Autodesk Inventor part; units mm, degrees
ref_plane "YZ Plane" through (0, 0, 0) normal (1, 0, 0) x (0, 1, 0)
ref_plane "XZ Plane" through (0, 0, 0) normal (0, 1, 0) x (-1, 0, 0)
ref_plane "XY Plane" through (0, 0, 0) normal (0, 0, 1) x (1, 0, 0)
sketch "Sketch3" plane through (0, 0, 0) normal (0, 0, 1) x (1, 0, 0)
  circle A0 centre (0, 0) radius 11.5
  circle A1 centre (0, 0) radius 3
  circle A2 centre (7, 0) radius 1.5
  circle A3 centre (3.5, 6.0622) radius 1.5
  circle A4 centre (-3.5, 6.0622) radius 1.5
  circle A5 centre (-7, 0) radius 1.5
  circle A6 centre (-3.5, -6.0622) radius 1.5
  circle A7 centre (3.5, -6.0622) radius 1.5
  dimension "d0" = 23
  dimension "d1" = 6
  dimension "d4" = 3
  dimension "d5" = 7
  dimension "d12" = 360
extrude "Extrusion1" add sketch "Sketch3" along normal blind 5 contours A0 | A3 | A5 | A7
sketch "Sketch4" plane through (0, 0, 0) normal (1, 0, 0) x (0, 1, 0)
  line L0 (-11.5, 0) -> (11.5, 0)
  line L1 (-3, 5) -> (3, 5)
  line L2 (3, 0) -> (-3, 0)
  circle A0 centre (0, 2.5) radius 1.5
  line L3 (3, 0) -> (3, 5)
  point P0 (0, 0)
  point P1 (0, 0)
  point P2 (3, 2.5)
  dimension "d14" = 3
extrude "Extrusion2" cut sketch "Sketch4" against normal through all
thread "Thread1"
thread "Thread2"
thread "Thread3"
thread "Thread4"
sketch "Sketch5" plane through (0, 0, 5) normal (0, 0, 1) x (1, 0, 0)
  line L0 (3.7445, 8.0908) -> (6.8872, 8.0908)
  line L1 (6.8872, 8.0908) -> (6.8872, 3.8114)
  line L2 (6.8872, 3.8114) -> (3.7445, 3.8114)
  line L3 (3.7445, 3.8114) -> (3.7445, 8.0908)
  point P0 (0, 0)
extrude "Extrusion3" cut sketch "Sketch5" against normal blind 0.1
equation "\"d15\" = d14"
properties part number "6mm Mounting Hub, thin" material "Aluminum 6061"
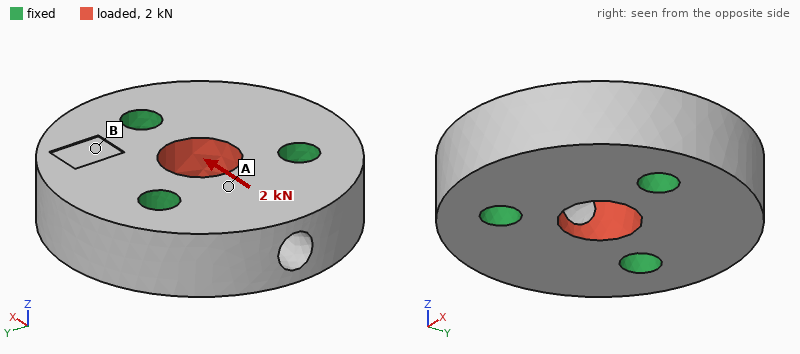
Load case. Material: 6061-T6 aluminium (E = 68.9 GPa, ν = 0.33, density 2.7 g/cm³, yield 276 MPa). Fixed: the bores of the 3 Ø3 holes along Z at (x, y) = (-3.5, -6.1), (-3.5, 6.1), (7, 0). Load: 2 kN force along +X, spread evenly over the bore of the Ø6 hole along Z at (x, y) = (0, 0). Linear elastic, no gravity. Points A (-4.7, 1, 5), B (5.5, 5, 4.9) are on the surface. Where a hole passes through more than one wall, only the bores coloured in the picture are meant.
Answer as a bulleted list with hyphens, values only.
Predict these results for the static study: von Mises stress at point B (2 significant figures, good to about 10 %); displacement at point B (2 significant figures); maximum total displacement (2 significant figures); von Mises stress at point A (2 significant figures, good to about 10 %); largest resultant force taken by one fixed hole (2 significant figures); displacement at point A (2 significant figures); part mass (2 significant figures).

- 7.0 MPa
- 0.81 µm
- 2.5 µm
- 20 MPa
- 710 N
- 1.8 µm
- 4.8 g
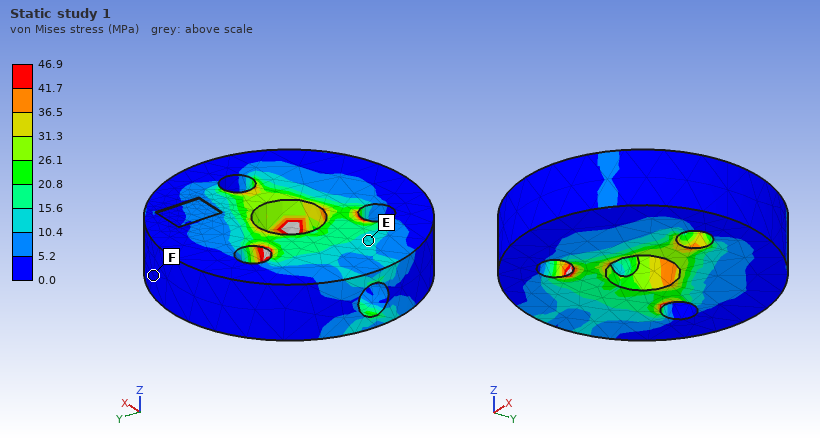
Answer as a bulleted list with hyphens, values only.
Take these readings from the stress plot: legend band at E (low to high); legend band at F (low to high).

- 10.4 to 15.6 MPa
- 0.0 to 5.2 MPa
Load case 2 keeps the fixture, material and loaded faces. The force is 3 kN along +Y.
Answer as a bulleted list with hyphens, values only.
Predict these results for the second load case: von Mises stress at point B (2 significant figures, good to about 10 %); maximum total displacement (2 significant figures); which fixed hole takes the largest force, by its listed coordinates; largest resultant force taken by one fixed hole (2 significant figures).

- 19 MPa
- 3.7 µm
- (7, 0)
- 1.1 kN
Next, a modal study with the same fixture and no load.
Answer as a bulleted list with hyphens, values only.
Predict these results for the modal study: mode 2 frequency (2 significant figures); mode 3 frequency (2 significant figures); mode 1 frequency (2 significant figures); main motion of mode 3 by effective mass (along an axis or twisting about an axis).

- 60 kHz
- 66 kHz
- 58 kHz
- along Z
